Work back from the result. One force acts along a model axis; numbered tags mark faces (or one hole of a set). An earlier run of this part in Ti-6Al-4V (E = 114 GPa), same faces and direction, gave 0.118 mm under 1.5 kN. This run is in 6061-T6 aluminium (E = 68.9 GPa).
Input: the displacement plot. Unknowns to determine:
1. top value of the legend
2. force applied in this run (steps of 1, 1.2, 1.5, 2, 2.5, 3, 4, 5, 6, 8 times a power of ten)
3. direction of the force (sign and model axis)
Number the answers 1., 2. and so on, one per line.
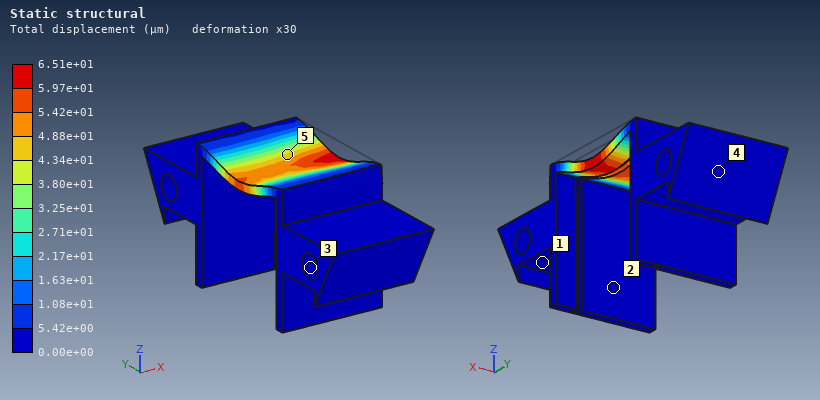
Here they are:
1. 6.51e+01 µm
2. 500 N
3. -Z
